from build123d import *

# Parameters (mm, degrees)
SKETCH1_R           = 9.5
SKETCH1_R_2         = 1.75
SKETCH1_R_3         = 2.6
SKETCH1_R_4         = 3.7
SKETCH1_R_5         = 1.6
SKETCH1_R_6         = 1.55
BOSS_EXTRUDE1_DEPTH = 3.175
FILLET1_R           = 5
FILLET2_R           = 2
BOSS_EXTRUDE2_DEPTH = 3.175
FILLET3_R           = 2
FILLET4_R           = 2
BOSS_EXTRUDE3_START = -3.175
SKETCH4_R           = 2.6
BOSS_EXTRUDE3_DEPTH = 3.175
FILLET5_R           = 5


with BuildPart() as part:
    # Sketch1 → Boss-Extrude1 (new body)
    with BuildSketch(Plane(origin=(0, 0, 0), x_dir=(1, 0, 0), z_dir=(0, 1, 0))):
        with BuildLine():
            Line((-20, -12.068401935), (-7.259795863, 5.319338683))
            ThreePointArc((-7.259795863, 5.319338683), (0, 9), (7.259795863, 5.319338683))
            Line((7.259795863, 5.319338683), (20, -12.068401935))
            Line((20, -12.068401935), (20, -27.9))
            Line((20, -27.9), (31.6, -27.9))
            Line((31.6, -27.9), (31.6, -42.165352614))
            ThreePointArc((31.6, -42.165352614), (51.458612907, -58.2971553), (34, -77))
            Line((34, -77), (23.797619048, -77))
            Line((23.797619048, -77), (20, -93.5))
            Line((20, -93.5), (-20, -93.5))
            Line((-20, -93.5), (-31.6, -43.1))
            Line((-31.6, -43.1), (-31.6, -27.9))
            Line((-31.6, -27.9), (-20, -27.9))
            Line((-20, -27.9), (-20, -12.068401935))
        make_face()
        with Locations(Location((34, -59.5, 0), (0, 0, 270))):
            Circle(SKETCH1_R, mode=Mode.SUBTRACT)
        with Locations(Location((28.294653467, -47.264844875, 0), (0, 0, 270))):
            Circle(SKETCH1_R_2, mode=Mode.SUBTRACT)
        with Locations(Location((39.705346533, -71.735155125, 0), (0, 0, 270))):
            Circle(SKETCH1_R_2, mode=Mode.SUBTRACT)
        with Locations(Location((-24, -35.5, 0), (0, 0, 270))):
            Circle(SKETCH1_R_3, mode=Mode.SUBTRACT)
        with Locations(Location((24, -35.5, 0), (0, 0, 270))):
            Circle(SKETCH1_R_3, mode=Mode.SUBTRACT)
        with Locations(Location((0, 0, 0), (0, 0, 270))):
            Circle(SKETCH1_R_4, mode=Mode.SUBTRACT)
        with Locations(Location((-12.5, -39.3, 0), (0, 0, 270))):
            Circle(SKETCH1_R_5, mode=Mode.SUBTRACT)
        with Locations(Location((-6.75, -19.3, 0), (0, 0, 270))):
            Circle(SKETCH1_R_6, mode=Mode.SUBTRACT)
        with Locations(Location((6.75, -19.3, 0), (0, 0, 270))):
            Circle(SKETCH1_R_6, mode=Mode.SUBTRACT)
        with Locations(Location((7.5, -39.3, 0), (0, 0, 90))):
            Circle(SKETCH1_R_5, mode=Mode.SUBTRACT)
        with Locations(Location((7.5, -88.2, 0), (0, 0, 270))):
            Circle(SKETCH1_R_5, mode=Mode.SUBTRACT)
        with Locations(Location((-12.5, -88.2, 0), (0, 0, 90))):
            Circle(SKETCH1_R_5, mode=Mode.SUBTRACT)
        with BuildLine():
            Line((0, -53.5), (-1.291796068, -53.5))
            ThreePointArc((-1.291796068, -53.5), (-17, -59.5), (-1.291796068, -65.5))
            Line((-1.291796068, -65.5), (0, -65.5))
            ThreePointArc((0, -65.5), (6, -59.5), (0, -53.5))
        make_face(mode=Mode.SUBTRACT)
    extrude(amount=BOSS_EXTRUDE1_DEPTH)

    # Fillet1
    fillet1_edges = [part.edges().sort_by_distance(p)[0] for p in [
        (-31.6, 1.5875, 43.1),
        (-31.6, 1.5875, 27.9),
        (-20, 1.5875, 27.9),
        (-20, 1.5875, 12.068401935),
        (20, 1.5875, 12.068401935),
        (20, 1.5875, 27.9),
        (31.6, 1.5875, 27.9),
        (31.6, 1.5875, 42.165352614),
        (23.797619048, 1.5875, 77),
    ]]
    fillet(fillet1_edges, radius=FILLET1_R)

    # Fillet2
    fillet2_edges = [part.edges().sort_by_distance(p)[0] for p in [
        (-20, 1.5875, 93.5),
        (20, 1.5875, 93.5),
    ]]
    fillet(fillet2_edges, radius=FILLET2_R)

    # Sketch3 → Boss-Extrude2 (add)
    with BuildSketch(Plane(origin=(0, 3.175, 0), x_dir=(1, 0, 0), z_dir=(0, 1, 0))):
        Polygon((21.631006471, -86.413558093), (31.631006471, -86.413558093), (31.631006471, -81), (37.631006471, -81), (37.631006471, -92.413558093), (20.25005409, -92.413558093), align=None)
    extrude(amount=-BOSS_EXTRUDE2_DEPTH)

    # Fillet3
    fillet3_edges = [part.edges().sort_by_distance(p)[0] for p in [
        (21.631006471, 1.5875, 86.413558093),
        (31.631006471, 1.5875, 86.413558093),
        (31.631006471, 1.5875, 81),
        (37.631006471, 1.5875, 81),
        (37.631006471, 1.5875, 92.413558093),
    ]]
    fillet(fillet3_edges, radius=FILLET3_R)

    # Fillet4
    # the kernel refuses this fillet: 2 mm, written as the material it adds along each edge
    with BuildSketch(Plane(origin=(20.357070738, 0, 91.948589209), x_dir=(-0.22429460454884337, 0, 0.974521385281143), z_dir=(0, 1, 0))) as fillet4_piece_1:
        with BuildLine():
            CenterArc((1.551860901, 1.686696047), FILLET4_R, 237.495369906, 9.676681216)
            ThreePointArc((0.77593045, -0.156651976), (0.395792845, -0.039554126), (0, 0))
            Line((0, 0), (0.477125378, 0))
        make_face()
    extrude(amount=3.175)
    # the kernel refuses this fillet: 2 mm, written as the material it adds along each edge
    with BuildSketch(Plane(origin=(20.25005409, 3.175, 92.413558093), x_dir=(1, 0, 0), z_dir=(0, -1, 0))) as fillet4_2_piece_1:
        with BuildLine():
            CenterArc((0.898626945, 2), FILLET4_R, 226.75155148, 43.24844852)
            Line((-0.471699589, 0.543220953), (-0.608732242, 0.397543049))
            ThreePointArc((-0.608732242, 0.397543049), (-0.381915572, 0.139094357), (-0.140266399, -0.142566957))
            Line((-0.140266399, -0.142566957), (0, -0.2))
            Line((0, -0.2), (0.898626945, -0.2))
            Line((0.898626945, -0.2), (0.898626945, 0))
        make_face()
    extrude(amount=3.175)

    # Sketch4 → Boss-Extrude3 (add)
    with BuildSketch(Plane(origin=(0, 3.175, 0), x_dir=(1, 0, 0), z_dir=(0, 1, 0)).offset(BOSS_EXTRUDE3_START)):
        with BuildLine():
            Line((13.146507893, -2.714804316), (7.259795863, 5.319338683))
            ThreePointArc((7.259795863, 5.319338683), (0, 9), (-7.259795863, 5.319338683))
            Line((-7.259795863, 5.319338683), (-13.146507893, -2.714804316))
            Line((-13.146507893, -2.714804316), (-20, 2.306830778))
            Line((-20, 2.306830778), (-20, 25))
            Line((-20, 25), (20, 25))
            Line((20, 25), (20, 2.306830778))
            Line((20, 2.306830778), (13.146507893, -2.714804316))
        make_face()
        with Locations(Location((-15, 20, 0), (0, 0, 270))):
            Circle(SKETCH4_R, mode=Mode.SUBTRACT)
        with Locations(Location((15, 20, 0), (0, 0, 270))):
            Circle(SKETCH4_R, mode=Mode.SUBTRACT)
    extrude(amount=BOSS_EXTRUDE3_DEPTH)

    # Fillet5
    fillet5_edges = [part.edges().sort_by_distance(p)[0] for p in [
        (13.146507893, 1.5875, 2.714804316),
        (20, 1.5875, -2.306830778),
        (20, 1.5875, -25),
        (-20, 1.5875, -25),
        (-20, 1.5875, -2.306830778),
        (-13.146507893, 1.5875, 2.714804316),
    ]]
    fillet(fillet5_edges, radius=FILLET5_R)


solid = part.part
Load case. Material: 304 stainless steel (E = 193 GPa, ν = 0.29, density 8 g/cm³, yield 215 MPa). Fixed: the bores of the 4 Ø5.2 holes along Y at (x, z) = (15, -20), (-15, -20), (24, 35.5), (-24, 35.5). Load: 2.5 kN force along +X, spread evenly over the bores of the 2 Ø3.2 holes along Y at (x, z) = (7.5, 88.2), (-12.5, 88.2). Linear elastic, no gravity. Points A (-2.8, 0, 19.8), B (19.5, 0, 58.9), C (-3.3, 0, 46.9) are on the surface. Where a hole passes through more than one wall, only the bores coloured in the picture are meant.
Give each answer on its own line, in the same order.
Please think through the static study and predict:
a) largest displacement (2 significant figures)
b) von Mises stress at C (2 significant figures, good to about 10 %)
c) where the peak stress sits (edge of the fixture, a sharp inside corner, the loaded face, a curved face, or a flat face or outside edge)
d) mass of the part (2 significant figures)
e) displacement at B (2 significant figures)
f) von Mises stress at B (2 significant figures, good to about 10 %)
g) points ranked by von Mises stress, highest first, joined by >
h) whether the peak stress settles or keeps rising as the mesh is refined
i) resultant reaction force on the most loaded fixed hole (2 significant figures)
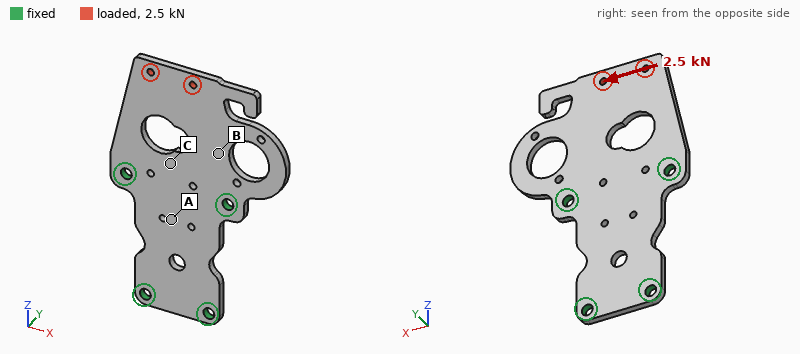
38 µm
33 MPa
edge of the fixture
140 g
12 µm
57 MPa
B > C > A
keeps rising
2.9 kN
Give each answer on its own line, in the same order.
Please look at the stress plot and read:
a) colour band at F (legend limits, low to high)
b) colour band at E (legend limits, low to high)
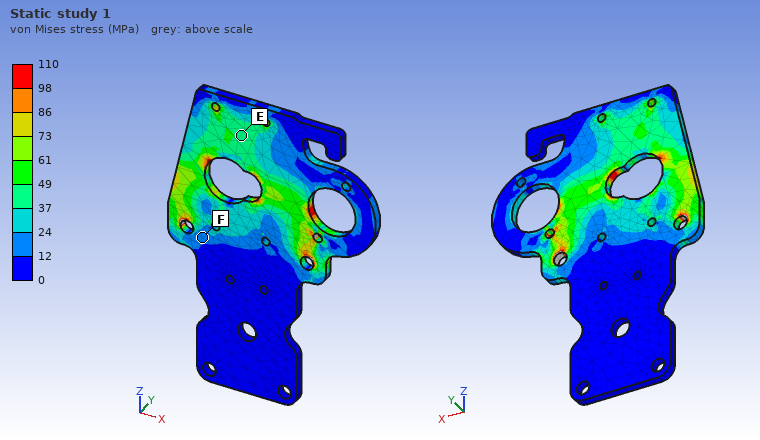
12 to 24 MPa
37 to 49 MPa
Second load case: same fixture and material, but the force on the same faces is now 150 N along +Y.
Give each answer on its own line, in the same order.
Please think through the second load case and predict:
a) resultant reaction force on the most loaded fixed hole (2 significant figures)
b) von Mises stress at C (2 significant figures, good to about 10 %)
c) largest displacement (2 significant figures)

93 N
30 MPa
0.37 mm
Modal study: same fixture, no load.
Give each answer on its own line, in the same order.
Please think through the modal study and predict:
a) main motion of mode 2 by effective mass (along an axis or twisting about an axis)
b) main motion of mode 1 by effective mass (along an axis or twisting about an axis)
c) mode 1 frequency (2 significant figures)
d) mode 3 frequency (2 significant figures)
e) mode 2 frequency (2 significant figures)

twisting about Z
along Y
710 Hz
2800 Hz
1600 Hz
